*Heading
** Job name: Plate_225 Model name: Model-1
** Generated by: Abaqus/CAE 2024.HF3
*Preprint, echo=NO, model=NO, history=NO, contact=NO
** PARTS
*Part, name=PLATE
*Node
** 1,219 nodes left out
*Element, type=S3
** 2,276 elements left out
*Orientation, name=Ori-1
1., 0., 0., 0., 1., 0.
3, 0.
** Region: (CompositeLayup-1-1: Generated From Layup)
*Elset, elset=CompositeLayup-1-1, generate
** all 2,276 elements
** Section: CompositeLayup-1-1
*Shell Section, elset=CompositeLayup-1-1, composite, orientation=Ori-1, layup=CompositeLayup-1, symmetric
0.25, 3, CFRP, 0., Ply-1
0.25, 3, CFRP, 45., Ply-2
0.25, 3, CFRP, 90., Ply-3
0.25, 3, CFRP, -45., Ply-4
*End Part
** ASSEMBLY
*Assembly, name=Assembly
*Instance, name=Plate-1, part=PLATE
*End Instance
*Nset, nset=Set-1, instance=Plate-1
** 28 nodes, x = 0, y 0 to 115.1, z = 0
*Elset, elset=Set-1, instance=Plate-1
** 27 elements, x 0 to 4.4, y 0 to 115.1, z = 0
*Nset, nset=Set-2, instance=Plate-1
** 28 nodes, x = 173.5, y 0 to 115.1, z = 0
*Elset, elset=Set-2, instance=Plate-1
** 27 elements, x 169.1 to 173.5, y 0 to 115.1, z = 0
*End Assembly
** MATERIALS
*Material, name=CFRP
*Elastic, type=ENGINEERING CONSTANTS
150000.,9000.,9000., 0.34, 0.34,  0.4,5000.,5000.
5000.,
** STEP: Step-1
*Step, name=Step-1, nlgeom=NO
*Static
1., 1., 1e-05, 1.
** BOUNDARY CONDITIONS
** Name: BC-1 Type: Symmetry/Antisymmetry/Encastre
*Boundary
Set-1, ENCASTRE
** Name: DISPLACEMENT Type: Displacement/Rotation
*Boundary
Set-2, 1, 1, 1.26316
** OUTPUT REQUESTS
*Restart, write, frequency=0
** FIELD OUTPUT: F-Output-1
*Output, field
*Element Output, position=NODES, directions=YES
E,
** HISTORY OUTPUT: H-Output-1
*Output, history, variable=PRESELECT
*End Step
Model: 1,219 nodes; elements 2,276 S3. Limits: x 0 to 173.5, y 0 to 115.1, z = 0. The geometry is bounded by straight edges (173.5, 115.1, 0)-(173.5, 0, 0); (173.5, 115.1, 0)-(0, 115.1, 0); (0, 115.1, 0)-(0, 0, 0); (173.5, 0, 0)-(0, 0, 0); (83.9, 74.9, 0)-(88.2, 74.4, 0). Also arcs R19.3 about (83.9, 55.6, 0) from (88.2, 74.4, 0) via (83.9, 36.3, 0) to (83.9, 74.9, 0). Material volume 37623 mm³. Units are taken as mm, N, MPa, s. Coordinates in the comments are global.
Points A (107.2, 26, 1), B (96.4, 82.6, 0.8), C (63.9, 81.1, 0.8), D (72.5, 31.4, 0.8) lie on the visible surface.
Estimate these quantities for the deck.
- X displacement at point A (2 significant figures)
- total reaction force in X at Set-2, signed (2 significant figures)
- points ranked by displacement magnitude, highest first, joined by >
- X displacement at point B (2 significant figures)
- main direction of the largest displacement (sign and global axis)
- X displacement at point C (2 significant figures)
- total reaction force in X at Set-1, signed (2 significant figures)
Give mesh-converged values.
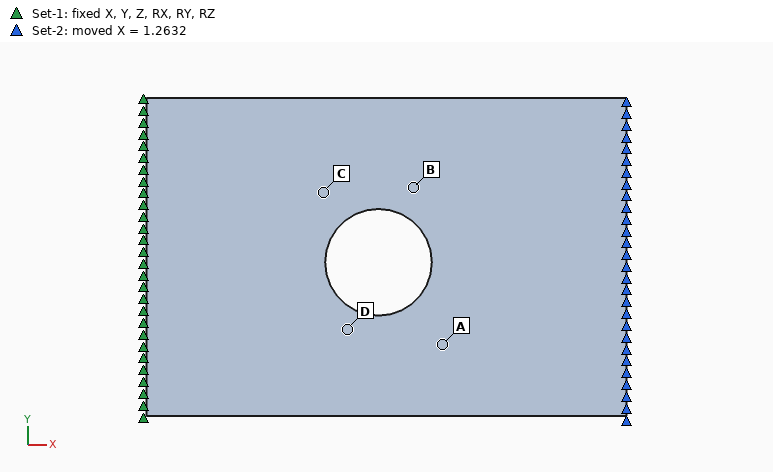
0.83 mm
80000 N
A > B > D > C
0.74 mm
+X
0.40 mm
-80000 N
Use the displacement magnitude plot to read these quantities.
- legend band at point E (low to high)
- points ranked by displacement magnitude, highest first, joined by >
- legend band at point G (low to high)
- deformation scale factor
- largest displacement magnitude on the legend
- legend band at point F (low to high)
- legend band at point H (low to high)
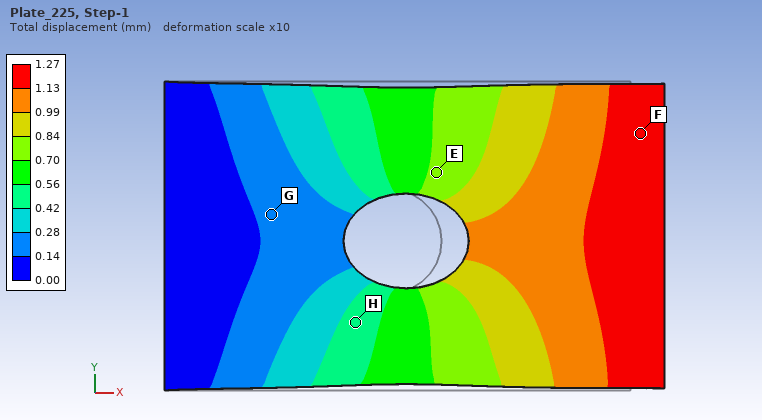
0.70 to 0.84 mm
F > E > H > G
0.14 to 0.28 mm
10
1.27 mm
1.13 to 1.27 mm
0.42 to 0.56 mm
